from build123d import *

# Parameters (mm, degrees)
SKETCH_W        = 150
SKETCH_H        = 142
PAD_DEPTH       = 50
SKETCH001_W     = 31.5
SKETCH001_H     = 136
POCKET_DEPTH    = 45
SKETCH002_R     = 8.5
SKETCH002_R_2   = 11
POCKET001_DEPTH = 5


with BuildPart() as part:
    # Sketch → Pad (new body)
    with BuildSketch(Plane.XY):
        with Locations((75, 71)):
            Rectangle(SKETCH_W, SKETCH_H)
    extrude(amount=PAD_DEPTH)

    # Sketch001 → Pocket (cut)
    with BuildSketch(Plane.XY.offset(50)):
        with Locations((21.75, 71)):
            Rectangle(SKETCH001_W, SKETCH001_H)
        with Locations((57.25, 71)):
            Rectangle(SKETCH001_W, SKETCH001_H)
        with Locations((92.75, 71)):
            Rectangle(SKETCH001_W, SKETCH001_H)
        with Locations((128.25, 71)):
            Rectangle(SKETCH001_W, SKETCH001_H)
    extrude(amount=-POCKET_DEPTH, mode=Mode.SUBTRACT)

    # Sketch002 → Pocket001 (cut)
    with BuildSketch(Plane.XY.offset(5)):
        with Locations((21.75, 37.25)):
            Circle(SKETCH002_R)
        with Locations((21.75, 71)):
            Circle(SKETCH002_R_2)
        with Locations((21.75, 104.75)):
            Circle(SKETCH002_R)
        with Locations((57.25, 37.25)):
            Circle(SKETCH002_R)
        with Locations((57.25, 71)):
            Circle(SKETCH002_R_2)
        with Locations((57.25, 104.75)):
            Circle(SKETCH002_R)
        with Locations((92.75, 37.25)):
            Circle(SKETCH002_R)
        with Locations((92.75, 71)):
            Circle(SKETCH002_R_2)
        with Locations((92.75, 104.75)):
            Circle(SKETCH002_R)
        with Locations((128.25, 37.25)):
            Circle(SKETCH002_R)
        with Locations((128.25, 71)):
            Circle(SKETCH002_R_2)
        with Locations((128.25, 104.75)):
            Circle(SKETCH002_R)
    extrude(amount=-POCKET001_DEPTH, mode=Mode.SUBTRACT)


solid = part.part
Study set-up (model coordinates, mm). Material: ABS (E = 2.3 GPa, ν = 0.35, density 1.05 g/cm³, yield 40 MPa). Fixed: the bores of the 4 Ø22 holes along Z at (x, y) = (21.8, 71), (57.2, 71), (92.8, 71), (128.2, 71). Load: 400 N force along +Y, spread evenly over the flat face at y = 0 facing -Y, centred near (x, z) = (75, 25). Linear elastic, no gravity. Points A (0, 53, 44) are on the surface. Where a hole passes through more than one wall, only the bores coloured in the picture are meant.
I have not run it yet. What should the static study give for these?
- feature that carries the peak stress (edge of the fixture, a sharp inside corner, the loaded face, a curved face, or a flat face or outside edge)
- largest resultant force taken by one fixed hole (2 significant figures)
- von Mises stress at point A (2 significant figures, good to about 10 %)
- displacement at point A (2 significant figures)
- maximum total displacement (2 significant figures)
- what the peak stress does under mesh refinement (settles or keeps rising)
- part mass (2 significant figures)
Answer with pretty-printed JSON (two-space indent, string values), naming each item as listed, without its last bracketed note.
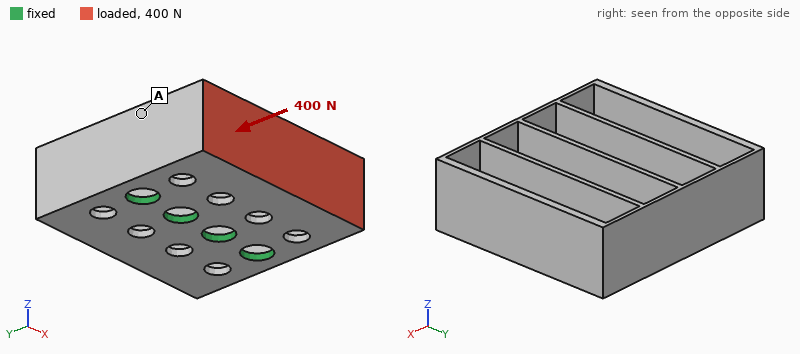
{
  "feature that carries the peak stress": "edge of the fixture",
  "largest resultant force taken by one fixed hole": "110 N",
  "von Mises stress at point A": "0.32 MPa",
  "displacement at point A": "0.10 mm",
  "maximum total displacement": "0.22 mm",
  "what the peak stress does under mesh refinement": "keeps rising",
  "part mass": "290 g"
}
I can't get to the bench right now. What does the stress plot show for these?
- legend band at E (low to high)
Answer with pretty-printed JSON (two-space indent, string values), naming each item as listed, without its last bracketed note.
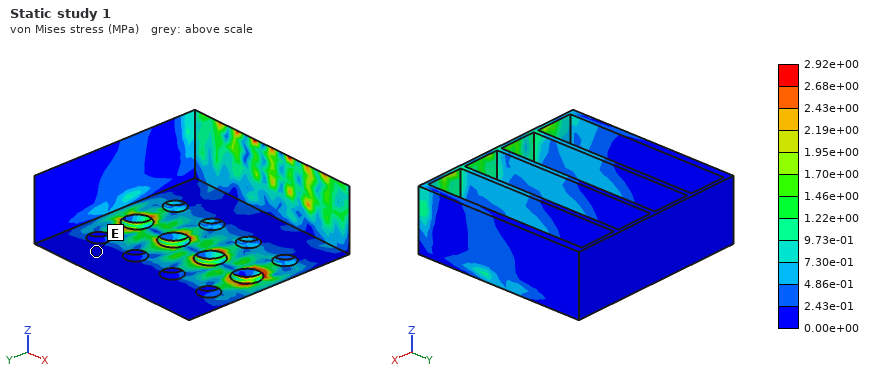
{
  "legend band at E": "0.00e+00 to 2.43e-01 MPa"
}
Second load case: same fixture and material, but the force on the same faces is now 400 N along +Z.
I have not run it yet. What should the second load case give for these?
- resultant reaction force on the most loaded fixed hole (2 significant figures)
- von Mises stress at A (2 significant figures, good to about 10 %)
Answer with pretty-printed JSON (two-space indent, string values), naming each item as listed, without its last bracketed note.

{
  "resultant reaction force on the most loaded fixed hole": "120 N",
  "von Mises stress at A": "1.2 MPa"
}
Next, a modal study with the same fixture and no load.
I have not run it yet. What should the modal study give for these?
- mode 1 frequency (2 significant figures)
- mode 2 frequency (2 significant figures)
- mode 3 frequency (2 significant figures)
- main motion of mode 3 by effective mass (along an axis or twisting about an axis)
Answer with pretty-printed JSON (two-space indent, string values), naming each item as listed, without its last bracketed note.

{
  "mode 1 frequency": "330 Hz",
  "mode 2 frequency": "370 Hz",
  "mode 3 frequency": "590 Hz",
  "main motion of mode 3 by effective mass": "along X"
}
